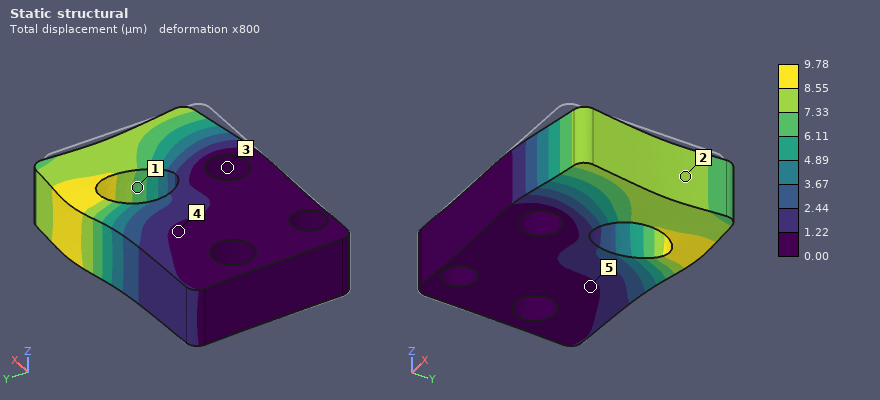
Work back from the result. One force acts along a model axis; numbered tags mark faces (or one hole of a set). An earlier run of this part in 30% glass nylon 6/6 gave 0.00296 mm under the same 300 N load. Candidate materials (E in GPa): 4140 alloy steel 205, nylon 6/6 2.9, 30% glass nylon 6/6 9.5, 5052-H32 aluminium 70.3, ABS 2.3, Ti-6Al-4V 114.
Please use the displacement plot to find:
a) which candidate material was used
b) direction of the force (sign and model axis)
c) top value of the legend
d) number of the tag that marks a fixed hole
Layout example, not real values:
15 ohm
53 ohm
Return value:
nylon 6/6
+Y
9.78 µm
3
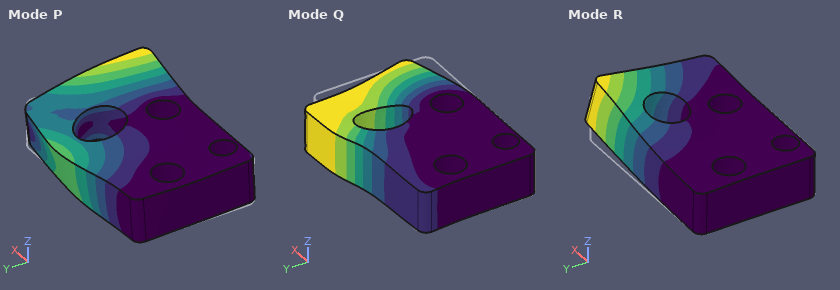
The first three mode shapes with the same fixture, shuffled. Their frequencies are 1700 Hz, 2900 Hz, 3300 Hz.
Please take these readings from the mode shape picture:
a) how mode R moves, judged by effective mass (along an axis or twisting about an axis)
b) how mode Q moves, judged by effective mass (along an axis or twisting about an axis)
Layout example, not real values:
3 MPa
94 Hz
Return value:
along Z
along Y
